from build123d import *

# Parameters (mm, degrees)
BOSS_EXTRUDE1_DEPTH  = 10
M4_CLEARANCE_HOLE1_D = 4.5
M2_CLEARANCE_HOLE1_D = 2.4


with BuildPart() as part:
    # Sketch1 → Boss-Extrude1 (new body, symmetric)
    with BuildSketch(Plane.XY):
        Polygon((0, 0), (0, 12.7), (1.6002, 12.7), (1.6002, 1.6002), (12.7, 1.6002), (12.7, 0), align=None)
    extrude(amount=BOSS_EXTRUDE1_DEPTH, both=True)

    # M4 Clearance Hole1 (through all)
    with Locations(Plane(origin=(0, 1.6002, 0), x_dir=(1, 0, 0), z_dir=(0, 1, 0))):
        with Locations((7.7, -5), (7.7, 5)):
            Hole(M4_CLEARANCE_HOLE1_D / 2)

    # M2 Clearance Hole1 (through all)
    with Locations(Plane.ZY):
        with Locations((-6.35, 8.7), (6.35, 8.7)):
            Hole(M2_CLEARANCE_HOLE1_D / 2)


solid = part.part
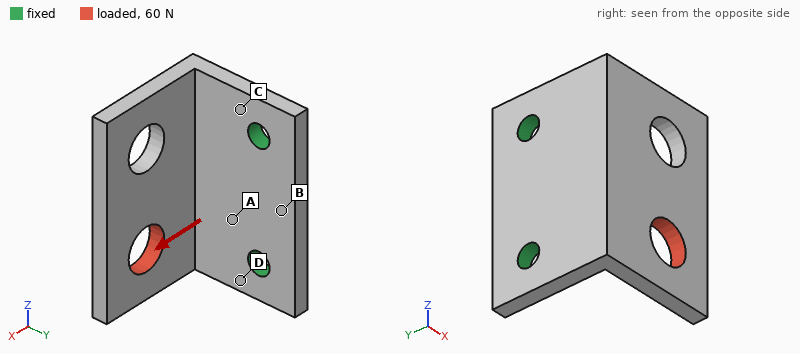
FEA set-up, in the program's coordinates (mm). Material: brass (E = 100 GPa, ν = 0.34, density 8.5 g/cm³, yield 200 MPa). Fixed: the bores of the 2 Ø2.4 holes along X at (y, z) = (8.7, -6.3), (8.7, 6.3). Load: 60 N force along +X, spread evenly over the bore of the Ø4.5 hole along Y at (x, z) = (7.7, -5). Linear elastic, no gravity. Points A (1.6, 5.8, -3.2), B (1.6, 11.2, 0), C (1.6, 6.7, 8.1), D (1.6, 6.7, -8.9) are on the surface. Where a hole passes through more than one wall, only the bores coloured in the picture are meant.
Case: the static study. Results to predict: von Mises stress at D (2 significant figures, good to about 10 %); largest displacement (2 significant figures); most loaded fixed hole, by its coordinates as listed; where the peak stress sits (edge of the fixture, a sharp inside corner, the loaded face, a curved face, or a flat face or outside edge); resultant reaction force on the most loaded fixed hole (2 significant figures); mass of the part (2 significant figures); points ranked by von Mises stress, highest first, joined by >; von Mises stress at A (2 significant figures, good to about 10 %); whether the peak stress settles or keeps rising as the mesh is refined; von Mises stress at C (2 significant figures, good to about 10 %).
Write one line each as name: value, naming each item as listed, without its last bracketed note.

von Mises stress at D: 53 MPa
largest displacement: 41 µm
most loaded fixed hole, by its coordinates as listed: (8.7, -6.3)
where the peak stress sits: edge of the fixture
resultant reaction force on the most loaded fixed hole: 51 N
mass of the part: 5.9 g
points ranked by von Mises stress, highest first, joined by >: D > A > C > B
von Mises stress at A: 34 MPa
whether the peak stress settles or keeps rising as the mesh is refined: keeps rising
von Mises stress at C: 24 MPa
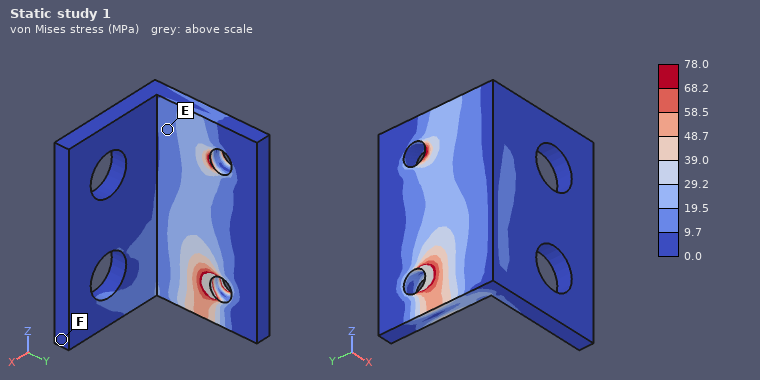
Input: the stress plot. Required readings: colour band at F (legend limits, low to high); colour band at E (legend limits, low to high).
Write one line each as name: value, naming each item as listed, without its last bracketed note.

colour band at F: 0.0 to 9.7 MPa
colour band at E: 9.7 to 19.5 MPa
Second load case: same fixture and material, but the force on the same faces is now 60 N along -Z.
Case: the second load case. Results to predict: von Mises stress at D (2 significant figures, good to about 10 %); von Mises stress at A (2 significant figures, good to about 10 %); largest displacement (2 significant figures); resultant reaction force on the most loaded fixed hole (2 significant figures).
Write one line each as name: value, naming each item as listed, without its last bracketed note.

von Mises stress at D: 22 MPa
von Mises stress at A: 18 MPa
largest displacement: 17 µm
resultant reaction force on the most loaded fixed hole: 53 N
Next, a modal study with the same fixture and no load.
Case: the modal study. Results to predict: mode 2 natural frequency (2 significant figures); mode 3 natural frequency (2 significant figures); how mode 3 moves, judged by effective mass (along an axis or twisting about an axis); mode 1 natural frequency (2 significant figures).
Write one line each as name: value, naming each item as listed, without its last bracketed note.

mode 2 natural frequency: 6100 Hz
mode 3 natural frequency: 9200 Hz
how mode 3 moves, judged by effective mass: along X
mode 1 natural frequency: 3300 Hz
